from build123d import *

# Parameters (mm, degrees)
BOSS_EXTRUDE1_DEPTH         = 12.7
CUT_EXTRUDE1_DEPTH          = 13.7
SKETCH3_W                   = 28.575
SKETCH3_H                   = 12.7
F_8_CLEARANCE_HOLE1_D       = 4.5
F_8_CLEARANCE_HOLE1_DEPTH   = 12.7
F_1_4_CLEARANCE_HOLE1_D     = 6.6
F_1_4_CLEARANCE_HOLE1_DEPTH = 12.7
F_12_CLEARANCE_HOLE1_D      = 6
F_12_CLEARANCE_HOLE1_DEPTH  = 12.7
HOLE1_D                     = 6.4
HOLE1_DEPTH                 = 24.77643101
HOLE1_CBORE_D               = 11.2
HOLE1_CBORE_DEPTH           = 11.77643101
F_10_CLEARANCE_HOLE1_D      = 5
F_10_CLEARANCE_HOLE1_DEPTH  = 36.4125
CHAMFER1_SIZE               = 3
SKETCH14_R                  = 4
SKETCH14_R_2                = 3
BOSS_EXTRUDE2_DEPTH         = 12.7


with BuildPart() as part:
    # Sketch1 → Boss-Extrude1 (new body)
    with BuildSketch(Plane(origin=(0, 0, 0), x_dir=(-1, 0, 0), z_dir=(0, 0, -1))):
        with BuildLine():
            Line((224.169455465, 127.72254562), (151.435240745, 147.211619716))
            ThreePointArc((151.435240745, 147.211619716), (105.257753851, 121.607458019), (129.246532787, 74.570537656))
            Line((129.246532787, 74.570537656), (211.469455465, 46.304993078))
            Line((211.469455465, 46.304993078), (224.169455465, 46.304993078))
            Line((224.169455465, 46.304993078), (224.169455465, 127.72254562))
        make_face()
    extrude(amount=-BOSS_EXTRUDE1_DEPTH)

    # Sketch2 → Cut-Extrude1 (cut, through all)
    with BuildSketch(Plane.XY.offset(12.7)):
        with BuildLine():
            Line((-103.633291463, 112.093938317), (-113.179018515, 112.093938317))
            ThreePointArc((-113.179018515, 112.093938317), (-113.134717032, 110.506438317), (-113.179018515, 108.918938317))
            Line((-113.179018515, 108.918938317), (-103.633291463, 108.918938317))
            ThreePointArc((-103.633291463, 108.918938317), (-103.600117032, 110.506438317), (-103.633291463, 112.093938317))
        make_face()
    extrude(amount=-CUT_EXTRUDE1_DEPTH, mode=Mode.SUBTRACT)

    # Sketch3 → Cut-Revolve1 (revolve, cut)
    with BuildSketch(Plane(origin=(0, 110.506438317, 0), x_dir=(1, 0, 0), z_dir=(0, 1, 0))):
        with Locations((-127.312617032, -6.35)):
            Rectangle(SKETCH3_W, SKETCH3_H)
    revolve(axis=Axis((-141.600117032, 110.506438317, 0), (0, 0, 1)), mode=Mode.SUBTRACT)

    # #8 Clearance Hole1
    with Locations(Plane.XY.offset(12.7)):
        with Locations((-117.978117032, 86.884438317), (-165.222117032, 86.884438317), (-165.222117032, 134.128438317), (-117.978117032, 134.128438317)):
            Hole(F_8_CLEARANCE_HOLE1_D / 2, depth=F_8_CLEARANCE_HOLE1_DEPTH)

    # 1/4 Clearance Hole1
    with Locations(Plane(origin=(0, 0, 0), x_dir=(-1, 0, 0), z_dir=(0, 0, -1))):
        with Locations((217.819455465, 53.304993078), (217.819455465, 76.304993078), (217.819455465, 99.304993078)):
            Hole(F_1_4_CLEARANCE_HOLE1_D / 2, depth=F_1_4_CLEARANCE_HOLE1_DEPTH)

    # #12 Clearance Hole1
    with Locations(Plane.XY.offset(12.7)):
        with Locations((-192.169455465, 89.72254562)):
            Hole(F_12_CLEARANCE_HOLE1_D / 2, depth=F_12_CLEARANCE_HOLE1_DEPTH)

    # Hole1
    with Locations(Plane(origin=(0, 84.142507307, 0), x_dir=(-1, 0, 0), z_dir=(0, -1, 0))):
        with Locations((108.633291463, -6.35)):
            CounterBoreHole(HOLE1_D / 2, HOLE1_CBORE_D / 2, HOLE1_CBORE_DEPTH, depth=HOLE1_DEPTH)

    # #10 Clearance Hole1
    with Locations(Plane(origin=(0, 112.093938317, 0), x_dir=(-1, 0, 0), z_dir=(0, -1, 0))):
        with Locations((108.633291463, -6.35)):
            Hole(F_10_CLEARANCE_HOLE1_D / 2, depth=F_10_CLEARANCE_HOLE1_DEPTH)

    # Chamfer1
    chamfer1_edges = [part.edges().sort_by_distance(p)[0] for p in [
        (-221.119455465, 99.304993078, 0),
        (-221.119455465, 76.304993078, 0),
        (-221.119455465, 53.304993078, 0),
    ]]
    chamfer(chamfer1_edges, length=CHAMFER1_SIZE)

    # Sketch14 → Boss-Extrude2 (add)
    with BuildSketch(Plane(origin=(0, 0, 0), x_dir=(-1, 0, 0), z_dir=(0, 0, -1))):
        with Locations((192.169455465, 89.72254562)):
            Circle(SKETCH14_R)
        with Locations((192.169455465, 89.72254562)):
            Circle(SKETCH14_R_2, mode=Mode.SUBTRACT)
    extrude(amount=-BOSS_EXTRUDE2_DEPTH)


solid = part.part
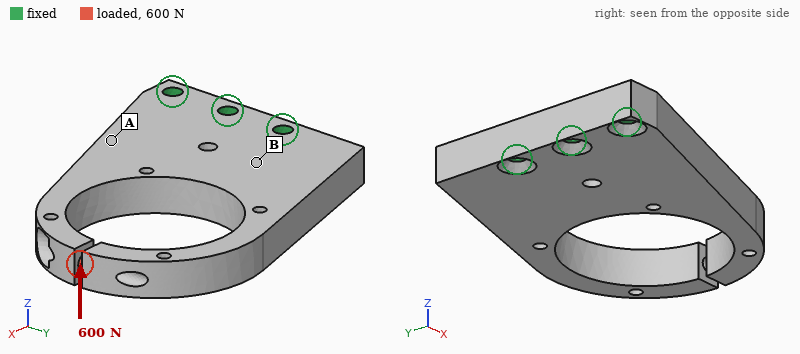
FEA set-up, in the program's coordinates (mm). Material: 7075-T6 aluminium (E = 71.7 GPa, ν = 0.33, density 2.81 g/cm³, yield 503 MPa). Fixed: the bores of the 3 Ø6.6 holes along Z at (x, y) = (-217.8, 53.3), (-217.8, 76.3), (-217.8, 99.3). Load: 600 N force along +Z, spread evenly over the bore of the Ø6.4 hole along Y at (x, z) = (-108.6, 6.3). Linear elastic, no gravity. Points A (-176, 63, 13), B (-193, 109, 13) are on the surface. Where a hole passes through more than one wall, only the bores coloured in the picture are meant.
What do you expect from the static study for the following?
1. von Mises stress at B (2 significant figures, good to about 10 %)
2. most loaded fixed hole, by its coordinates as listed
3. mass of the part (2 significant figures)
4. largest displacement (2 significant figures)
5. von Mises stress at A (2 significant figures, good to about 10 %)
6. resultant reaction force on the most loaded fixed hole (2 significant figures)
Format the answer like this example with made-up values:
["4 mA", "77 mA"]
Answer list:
["18 MPa", "(-217.8, 76.3)", "220 g", "0.89 mm", "39 MPa", "480 N"]
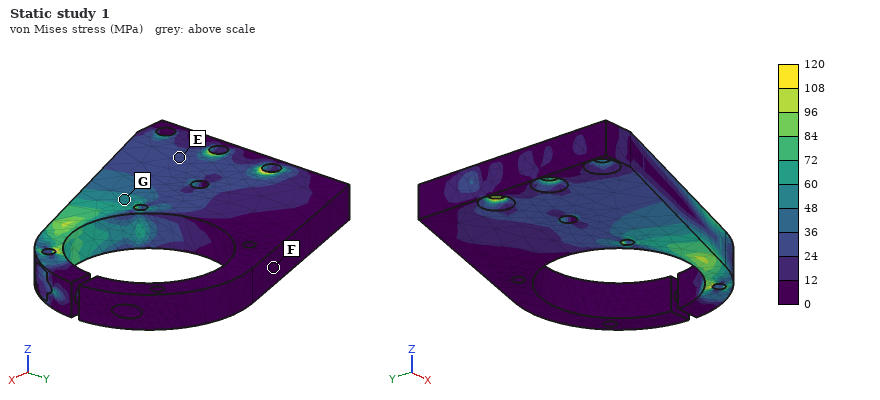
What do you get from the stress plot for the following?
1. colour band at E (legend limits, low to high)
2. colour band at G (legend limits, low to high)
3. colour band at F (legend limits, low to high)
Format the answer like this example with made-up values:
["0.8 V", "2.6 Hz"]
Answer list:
["24 to 36 MPa", "48 to 60 MPa", "0 to 12 MPa"]
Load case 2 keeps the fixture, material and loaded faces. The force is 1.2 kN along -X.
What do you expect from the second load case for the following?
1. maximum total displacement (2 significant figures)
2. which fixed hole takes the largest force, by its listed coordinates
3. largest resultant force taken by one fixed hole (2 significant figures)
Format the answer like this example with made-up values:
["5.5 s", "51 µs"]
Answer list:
["0.69 mm", "(-217.8, 99.3)", "1.1 kN"]
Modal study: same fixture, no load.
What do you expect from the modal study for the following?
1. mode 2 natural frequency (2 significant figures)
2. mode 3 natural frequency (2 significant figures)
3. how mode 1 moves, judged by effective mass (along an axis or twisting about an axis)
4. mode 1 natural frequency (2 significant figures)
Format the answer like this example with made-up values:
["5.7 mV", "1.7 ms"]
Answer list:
["1500 Hz", "1600 Hz", "along Z", "1000 Hz"]
